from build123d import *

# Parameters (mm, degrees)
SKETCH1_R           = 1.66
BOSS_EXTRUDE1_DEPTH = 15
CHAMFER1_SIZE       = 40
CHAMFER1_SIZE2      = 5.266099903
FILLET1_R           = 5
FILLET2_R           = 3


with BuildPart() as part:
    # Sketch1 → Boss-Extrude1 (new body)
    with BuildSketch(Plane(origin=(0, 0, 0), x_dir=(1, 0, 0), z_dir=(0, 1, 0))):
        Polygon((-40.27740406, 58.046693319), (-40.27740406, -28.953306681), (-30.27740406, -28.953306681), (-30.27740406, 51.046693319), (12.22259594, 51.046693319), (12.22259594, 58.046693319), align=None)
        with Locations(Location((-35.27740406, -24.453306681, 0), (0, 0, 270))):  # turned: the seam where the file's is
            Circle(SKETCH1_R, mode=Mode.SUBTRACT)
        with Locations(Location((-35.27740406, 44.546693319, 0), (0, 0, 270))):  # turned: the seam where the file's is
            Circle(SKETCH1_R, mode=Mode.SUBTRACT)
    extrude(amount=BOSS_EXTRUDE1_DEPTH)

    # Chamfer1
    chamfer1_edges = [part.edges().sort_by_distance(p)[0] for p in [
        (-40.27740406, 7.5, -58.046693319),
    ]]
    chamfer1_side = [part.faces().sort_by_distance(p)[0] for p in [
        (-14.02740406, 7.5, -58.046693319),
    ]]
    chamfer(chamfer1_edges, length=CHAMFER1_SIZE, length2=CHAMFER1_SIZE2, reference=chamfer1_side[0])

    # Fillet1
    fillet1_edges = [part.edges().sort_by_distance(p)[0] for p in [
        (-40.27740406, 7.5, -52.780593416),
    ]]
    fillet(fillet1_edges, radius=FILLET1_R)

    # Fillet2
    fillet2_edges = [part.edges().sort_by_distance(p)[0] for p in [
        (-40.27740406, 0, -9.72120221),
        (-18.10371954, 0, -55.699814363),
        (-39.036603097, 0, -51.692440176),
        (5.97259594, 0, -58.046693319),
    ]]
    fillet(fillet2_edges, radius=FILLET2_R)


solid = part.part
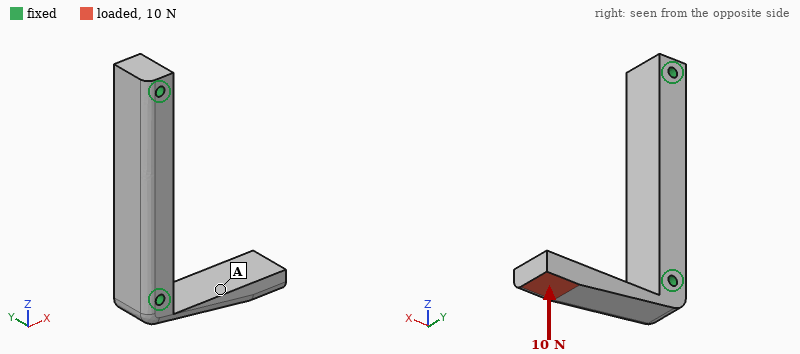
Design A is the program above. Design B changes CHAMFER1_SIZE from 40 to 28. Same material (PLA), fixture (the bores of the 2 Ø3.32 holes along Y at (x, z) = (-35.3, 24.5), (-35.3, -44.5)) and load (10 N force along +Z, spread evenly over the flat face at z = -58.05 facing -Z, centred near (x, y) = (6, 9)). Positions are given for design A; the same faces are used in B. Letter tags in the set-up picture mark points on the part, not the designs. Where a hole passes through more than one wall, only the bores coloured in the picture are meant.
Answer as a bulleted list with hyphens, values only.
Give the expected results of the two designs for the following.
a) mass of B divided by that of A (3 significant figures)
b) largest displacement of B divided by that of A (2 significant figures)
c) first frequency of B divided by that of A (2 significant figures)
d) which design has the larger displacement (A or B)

- 1.03
- 0.50
- 1.2
- A
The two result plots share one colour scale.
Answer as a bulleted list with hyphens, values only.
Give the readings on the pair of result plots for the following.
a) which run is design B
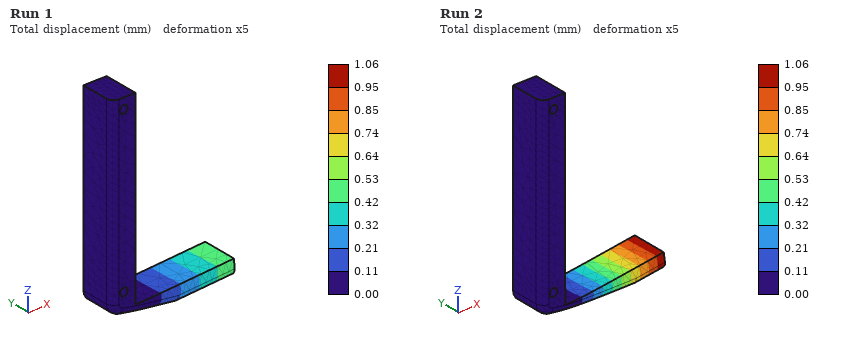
- Run 1
